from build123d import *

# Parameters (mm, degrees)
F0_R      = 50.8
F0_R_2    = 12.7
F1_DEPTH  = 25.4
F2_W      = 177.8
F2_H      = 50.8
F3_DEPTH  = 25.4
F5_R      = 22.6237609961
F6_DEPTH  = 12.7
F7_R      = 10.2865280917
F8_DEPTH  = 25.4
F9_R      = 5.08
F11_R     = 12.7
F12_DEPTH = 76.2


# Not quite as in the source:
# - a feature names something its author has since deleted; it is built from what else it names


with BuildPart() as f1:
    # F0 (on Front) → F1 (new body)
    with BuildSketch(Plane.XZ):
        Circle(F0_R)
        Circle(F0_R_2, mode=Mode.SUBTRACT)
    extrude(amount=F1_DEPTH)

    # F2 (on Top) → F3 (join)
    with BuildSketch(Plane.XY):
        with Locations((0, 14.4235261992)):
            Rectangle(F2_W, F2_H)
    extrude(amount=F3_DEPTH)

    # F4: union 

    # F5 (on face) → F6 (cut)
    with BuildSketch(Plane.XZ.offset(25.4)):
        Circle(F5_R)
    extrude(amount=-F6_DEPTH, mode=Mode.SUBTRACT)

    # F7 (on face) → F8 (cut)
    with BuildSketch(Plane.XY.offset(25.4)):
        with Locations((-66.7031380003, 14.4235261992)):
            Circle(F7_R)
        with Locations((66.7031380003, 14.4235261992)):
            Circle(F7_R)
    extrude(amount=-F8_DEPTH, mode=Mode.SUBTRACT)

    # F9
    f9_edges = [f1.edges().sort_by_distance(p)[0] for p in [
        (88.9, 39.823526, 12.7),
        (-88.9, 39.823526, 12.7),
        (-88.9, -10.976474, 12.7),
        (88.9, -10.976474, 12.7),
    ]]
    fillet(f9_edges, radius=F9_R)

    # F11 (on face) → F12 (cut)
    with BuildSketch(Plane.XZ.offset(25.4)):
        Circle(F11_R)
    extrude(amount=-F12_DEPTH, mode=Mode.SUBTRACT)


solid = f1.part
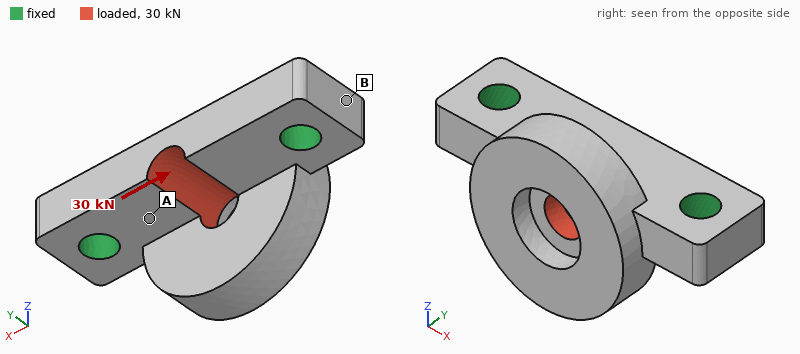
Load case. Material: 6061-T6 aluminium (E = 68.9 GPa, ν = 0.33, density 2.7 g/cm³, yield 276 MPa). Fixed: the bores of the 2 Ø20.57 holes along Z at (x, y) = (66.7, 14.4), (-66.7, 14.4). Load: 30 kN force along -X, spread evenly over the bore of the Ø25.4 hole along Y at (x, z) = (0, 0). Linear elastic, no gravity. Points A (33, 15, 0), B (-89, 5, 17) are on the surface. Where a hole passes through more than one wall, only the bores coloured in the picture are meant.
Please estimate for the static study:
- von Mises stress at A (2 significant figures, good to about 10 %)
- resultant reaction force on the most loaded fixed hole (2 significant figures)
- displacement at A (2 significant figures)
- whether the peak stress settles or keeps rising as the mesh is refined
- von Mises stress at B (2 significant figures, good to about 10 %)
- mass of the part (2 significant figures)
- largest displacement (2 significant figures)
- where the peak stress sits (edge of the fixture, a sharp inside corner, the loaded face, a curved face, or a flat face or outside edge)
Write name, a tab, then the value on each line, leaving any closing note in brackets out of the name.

von Mises stress at A	15 MPa
resultant reaction force on the most loaded fixed hole	15 kN
displacement at A	5.1 µm
whether the peak stress settles or keeps rising as the mesh is refined	keeps rising
von Mises stress at B	4.0 MPa
mass of the part	960 g
largest displacement	15 µm
where the peak stress sits	edge of the fixture
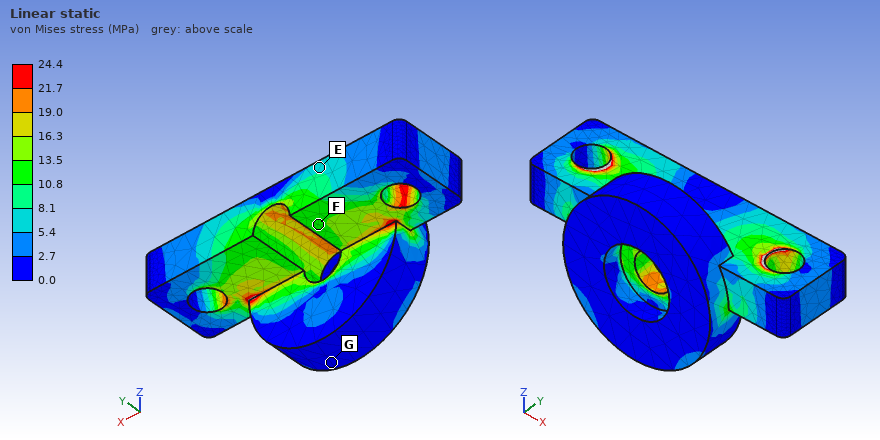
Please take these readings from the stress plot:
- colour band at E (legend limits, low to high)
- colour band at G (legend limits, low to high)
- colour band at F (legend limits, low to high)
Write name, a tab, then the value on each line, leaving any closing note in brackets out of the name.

colour band at E	5.4 to 8.1 MPa
colour band at G	0.0 to 2.7 MPa
colour band at F	10.8 to 13.5 MPa
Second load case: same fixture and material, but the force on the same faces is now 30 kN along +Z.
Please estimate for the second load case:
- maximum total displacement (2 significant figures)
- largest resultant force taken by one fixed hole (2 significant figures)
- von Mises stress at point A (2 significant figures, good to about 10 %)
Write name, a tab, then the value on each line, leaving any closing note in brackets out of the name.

maximum total displacement	72 µm
largest resultant force taken by one fixed hole	16 kN
von Mises stress at point A	21 MPa
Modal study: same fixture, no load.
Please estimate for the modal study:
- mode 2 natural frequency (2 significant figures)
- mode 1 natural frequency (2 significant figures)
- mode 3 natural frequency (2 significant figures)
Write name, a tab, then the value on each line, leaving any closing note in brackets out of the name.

mode 2 natural frequency	5800 Hz
mode 1 natural frequency	2900 Hz
mode 3 natural frequency	6900 Hz
